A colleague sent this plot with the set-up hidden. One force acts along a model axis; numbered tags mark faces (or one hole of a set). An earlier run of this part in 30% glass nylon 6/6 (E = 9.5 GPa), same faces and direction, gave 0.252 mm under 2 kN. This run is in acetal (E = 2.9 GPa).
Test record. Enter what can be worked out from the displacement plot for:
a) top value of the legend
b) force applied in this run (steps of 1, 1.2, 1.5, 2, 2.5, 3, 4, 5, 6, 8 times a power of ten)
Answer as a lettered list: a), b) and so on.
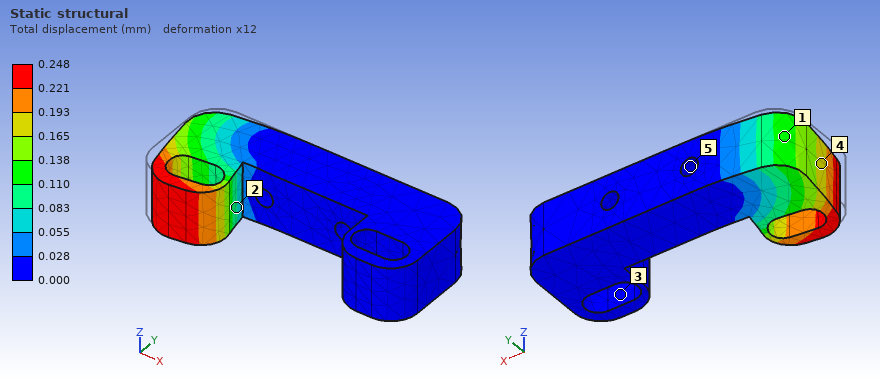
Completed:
a) 0.248 mm
b) 600 N
